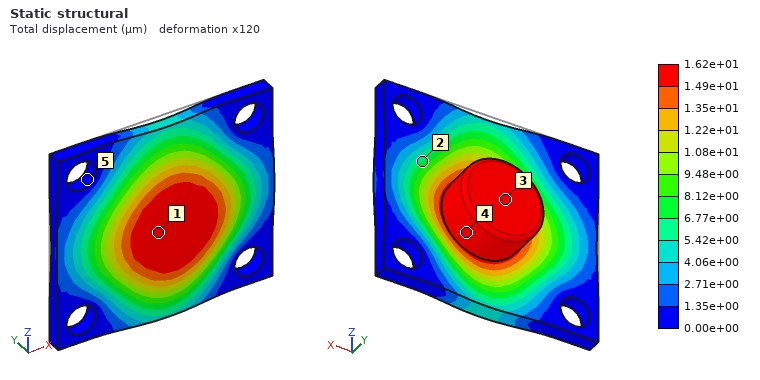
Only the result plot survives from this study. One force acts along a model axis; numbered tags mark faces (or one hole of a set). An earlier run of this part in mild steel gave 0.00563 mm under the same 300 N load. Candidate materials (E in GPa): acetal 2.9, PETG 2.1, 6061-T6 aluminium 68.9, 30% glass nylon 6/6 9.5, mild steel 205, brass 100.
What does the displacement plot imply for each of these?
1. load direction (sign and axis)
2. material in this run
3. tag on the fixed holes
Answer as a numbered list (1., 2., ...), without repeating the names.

1. -Y
2. 6061-T6 aluminium
3. 5
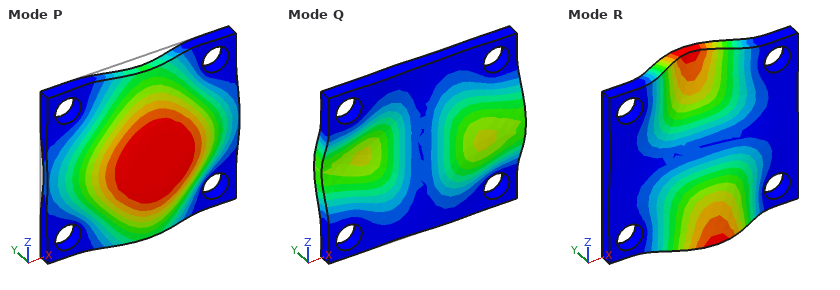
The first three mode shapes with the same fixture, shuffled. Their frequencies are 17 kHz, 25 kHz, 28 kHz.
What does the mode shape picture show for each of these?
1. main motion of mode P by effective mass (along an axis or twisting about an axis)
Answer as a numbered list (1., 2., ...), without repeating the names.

1. along Y
